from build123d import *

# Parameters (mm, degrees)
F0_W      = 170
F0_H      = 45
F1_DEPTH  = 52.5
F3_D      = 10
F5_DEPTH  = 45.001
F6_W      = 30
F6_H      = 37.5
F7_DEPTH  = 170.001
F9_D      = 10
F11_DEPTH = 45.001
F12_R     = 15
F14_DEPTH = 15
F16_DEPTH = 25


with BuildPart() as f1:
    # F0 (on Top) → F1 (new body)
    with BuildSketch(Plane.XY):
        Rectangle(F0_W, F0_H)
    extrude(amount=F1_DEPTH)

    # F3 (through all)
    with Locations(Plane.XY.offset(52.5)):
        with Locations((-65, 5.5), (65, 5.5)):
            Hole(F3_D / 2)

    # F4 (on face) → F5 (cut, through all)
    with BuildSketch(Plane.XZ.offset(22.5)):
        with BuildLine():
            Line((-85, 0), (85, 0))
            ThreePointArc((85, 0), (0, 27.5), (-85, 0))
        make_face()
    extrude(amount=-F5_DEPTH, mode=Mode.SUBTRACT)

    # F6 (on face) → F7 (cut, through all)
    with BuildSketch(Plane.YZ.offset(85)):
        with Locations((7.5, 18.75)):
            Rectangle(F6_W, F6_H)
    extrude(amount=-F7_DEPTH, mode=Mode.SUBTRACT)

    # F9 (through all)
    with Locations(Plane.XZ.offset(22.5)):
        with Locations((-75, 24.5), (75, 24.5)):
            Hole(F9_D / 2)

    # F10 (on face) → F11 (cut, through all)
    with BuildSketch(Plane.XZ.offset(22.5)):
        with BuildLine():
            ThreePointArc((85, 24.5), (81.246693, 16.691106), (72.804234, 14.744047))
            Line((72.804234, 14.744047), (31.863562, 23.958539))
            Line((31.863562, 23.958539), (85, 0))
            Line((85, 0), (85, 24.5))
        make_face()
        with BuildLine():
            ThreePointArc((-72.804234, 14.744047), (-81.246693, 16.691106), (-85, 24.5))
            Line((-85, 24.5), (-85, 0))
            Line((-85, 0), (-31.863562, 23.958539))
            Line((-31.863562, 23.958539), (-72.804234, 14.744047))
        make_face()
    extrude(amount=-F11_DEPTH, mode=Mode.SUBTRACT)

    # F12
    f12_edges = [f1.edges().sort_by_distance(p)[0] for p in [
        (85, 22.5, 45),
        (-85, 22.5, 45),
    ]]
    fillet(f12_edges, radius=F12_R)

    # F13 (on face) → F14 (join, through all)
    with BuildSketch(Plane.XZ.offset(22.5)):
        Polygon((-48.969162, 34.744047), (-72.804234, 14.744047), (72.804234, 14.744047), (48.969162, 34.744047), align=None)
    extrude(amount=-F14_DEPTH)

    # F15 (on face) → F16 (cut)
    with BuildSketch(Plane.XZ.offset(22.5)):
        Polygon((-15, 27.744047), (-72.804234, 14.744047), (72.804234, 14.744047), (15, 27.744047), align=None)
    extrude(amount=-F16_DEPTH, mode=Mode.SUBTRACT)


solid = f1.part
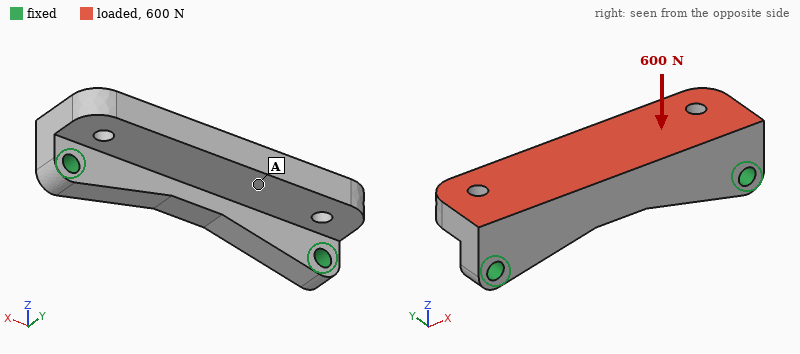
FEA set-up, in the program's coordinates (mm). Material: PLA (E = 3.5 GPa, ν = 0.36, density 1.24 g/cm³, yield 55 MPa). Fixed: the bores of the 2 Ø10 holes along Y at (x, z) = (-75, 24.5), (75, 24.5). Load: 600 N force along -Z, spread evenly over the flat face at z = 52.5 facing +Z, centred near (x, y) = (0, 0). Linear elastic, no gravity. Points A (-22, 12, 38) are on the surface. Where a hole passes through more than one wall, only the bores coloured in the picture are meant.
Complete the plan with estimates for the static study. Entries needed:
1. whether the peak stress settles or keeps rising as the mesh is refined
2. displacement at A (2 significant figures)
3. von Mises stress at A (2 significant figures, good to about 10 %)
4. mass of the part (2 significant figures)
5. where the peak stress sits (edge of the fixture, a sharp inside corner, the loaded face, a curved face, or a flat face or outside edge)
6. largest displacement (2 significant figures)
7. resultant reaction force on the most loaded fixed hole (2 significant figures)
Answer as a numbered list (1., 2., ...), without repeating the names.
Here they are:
1. keeps rising
2. 0.14 mm
3. 0.86 MPa
4. 180 g
5. edge of the fixture
6. 0.20 mm
7. 390 N
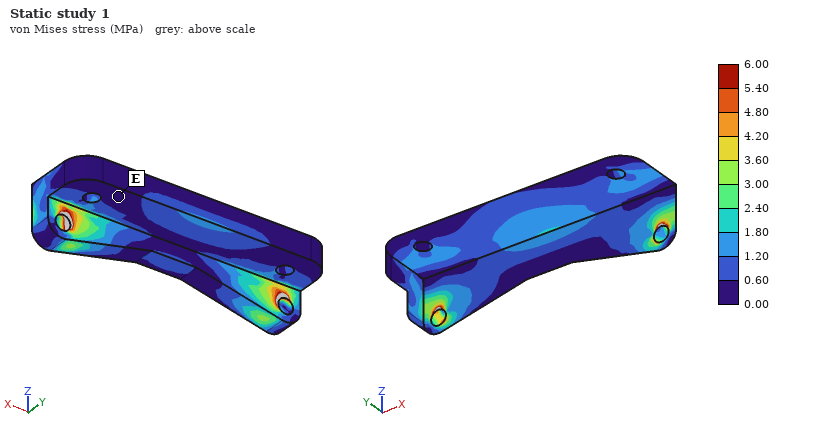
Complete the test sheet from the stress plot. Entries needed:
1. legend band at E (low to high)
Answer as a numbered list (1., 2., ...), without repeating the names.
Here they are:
1. 0.00 to 0.60 MPa
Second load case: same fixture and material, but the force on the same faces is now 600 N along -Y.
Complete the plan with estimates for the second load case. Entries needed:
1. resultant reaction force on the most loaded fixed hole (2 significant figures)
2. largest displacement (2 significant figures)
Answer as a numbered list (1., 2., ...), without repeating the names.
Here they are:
1. 310 N
2. 0.21 mm
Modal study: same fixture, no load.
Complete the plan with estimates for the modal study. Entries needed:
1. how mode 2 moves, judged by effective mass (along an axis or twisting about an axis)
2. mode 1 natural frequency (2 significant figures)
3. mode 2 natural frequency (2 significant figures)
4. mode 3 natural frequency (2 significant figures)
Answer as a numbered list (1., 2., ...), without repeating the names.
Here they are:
1. along Y
2. 860 Hz
3. 1600 Hz
4. 1700 Hz
